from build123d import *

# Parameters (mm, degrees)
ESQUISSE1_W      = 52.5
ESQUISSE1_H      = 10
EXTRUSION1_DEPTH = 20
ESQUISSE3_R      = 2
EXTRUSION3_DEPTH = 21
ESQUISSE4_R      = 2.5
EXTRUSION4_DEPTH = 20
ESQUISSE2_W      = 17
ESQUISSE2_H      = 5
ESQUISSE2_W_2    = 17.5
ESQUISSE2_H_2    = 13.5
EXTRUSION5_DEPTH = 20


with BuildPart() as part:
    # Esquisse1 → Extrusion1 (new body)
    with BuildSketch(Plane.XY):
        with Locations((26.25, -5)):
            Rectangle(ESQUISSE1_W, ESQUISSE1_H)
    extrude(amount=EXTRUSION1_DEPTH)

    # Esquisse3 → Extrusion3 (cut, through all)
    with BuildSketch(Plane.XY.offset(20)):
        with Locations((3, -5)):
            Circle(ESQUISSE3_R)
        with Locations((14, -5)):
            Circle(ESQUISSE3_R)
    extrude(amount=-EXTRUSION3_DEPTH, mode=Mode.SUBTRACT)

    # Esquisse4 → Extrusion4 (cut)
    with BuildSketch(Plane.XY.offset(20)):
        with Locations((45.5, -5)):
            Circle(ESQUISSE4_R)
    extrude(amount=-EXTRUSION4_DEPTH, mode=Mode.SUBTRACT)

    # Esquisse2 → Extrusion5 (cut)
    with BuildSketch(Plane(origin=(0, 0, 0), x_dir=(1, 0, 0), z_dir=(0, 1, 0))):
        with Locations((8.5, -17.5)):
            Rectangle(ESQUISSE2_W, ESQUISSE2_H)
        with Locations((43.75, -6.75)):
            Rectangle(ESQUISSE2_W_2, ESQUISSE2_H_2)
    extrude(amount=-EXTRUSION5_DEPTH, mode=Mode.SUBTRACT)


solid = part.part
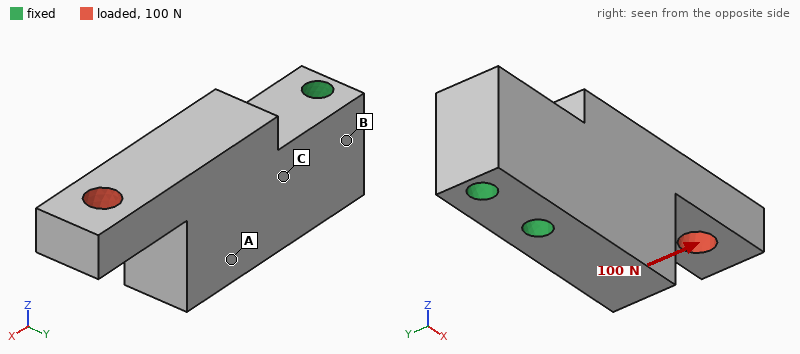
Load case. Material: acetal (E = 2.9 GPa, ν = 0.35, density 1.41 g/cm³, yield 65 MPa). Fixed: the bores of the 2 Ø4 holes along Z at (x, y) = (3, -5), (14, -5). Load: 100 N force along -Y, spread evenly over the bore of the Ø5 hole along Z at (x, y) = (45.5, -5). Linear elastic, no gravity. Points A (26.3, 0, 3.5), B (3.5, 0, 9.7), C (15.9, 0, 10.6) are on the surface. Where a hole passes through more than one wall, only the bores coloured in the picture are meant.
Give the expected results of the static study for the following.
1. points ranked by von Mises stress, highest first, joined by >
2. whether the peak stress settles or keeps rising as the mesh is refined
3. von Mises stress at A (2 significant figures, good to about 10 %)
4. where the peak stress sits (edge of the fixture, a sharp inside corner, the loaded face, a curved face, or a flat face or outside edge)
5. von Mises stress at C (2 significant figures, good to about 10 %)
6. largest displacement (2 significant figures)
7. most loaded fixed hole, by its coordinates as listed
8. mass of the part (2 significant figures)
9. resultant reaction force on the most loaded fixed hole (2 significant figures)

C > A > B
keeps rising
5.3 MPa
edge of the fixture
10 MPa
0.60 mm
(14, -5)
9.6 g
200 N
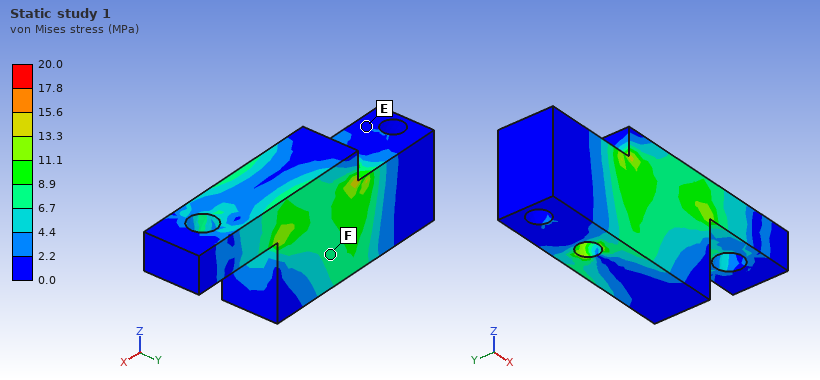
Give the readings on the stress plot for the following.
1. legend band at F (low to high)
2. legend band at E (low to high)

6.7 to 8.9 MPa
0.0 to 2.2 MPa
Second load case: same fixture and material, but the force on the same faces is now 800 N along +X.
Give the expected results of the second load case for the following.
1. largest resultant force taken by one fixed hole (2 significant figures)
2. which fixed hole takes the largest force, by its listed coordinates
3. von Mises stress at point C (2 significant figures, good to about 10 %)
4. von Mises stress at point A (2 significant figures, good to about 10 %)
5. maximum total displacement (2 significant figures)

740 N
(14, -5)
4.7 MPa
4.0 MPa
0.42 mm
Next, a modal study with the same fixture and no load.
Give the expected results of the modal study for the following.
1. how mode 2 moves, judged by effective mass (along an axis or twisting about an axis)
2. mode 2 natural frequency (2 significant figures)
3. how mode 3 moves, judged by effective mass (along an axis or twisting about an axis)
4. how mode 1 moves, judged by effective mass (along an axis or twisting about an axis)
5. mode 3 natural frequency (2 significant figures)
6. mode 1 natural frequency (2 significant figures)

along Z
2600 Hz
along Z
along Y
5800 Hz
1900 Hz
